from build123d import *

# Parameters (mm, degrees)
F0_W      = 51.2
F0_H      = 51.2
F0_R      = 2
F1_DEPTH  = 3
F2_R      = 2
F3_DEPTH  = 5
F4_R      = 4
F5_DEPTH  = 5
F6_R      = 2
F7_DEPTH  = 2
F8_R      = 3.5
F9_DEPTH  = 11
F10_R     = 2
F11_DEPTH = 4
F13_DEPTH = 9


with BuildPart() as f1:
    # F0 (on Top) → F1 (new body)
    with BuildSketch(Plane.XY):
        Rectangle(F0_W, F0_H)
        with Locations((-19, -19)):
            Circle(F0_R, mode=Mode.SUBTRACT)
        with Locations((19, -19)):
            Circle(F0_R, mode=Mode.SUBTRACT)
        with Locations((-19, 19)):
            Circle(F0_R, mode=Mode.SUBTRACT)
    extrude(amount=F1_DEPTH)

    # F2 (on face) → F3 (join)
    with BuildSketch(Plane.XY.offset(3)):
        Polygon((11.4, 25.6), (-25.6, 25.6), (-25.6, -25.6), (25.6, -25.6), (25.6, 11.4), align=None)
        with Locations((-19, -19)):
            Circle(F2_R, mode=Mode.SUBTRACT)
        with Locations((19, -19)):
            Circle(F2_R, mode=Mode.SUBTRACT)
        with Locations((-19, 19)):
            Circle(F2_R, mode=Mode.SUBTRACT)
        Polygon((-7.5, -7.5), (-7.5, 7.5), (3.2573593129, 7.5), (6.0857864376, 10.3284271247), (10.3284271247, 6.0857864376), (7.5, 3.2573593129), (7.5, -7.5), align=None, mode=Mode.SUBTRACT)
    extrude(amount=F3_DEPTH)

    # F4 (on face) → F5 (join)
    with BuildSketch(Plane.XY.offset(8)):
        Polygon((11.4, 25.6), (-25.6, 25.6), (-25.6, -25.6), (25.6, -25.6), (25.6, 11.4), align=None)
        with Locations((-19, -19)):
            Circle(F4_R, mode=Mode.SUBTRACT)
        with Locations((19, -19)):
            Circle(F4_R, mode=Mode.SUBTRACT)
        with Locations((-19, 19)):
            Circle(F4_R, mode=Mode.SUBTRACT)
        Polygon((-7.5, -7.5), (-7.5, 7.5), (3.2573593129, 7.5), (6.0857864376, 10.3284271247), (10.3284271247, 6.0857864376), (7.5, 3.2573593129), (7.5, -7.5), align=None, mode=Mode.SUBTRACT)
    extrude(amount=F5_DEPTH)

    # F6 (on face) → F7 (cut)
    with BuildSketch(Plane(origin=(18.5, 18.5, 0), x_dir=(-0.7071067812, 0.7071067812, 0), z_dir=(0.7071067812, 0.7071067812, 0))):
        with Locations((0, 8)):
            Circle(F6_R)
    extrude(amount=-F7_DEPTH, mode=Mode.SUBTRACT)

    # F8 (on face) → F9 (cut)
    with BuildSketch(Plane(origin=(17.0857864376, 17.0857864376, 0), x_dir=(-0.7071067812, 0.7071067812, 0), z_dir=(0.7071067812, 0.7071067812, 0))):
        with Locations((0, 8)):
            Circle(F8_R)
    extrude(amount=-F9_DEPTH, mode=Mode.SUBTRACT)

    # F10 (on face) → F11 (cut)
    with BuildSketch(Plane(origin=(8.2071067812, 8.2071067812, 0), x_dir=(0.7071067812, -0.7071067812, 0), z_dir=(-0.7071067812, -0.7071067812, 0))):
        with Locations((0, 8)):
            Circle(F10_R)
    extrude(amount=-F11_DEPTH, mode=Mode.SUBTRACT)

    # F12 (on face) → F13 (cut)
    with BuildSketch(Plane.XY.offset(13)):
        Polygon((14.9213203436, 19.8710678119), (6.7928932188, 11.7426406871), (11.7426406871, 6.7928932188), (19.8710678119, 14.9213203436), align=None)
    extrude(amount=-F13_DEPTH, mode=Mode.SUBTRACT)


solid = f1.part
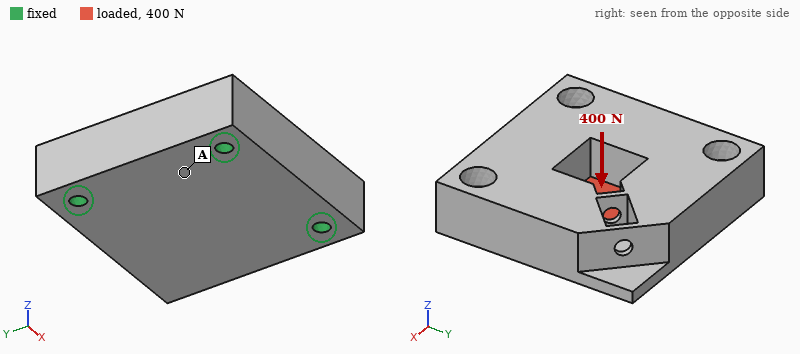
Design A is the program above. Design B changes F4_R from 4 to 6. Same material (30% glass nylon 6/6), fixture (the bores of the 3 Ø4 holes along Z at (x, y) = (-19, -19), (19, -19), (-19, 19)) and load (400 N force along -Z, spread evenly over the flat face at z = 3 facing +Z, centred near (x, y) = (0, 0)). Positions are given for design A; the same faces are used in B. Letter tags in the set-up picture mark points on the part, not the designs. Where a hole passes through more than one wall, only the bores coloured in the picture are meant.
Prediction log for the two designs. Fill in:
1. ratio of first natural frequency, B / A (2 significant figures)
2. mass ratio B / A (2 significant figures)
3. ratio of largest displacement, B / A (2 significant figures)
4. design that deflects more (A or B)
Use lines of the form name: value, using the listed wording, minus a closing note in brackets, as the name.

ratio of first natural frequency, B / A: 0.96
mass ratio B / A: 0.97
ratio of largest displacement, B / A: 1.1
design that deflects more: B
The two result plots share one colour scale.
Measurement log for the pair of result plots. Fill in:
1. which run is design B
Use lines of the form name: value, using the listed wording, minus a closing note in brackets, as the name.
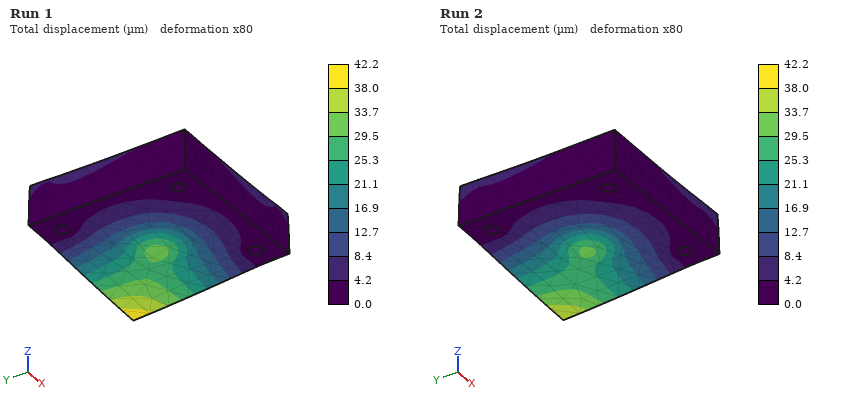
which run is design B: Run 1
